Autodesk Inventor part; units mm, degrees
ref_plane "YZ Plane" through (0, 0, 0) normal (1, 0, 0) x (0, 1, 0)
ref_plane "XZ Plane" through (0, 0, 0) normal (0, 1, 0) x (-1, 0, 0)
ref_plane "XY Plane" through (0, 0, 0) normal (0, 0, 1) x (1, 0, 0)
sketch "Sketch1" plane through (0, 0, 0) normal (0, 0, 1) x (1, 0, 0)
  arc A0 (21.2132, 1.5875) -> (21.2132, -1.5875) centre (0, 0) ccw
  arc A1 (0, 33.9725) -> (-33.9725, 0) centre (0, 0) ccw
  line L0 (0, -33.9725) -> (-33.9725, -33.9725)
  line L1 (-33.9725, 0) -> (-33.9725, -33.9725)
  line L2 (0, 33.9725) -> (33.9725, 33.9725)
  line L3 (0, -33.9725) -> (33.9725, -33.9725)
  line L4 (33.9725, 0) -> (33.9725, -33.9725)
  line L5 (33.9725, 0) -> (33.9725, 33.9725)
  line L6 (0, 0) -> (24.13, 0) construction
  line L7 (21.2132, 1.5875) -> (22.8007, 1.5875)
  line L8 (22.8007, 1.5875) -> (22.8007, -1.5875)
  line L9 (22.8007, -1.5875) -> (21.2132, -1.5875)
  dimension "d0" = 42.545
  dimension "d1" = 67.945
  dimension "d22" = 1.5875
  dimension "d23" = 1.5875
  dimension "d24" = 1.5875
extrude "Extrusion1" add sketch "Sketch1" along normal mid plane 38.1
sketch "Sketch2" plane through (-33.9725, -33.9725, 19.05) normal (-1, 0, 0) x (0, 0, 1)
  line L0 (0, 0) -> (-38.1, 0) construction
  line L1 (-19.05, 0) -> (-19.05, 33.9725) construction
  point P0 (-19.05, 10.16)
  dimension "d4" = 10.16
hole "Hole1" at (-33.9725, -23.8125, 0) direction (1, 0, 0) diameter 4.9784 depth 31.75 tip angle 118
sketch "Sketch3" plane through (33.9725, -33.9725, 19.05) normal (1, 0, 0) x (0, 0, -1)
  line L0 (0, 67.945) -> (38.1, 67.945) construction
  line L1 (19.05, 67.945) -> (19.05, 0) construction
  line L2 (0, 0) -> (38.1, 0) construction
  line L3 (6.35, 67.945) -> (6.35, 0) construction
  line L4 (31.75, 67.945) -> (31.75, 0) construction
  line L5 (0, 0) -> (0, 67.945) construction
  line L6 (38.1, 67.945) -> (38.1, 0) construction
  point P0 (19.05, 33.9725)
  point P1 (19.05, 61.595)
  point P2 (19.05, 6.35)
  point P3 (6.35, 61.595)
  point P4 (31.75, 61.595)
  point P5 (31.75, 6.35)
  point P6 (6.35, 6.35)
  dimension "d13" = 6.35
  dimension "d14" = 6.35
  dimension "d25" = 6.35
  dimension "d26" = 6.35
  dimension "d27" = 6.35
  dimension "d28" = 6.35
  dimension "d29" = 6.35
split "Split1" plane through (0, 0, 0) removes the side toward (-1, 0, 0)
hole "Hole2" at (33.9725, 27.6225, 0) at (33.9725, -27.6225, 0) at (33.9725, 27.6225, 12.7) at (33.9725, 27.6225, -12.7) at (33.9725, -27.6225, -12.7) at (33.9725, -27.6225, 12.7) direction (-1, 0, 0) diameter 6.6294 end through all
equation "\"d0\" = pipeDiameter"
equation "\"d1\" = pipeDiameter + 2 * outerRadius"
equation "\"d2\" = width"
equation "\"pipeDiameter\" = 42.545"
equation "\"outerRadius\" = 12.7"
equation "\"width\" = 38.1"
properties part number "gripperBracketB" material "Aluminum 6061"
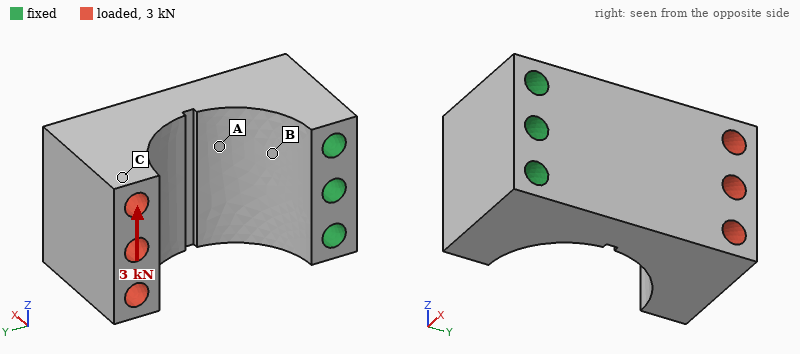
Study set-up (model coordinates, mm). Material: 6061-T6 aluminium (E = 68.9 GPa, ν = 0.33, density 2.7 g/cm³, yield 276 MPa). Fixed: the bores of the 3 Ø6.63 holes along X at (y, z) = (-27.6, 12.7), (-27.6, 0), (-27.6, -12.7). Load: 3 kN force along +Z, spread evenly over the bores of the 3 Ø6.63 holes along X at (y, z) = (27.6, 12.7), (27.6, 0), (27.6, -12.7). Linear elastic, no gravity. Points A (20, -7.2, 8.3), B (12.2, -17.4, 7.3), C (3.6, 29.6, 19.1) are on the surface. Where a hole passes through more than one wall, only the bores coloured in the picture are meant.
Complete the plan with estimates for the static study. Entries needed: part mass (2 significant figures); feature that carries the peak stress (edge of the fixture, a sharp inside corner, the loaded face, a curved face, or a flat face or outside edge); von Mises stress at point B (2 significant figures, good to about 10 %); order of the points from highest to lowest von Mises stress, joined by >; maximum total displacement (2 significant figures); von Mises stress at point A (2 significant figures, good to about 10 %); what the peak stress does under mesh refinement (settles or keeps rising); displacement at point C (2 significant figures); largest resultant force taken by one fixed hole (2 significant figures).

140 g
edge of the fixture
15 MPa
A > B > C
92 µm
39 MPa
keeps rising
84 µm
5.7 kN
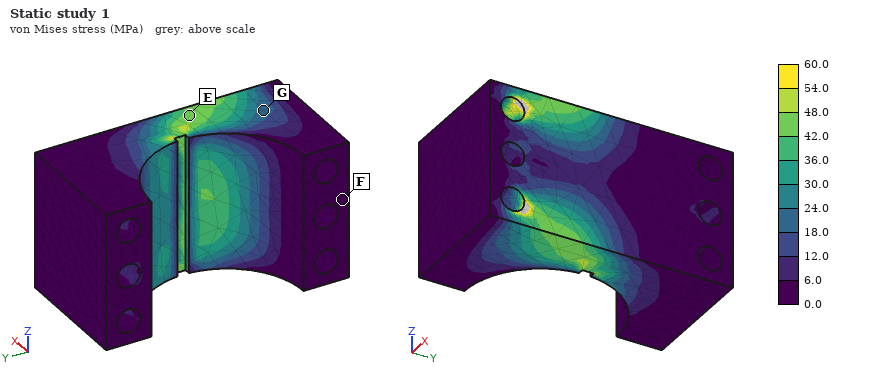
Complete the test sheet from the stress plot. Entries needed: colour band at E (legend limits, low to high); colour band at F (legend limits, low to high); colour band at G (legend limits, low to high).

42.0 to 48.0 MPa
0.0 to 6.0 MPa
18.0 to 24.0 MPa
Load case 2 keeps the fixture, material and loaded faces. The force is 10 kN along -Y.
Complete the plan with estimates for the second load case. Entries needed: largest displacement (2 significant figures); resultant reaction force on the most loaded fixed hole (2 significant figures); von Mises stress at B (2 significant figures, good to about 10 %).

0.32 mm
3.7 kN
18 MPa
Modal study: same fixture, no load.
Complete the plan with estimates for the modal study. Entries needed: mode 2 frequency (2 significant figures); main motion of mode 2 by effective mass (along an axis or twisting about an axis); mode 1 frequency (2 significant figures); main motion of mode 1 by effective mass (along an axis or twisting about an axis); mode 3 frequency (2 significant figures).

4800 Hz
along Z
2700 Hz
along X
7900 Hz
